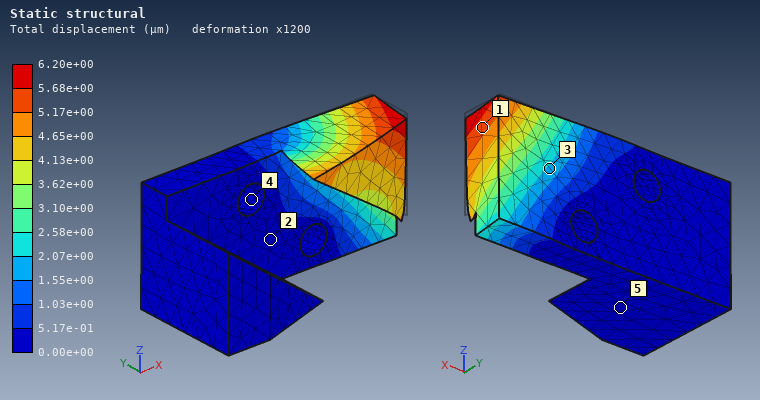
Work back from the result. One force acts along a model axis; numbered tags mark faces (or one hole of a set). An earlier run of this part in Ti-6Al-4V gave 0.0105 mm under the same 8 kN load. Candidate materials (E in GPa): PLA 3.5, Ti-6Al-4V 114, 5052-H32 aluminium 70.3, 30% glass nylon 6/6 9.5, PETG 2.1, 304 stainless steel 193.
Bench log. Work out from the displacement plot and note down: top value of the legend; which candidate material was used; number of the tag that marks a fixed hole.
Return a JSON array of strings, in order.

["6.20e+00 µm", "304 stainless steel", "4"]
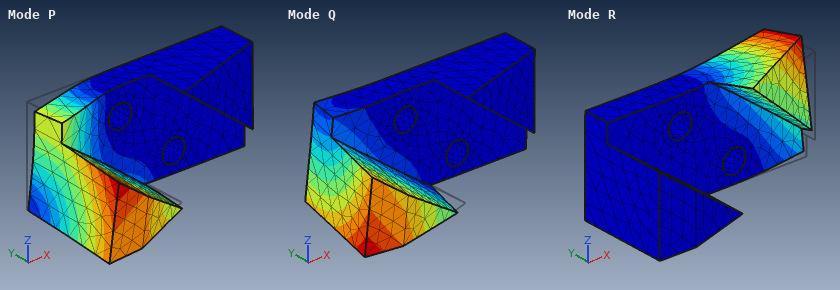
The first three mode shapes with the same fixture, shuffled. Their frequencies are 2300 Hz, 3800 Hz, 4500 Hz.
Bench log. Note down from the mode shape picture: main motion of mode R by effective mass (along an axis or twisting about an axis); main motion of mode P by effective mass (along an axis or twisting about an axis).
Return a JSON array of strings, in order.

["along Y", "along Z"]
